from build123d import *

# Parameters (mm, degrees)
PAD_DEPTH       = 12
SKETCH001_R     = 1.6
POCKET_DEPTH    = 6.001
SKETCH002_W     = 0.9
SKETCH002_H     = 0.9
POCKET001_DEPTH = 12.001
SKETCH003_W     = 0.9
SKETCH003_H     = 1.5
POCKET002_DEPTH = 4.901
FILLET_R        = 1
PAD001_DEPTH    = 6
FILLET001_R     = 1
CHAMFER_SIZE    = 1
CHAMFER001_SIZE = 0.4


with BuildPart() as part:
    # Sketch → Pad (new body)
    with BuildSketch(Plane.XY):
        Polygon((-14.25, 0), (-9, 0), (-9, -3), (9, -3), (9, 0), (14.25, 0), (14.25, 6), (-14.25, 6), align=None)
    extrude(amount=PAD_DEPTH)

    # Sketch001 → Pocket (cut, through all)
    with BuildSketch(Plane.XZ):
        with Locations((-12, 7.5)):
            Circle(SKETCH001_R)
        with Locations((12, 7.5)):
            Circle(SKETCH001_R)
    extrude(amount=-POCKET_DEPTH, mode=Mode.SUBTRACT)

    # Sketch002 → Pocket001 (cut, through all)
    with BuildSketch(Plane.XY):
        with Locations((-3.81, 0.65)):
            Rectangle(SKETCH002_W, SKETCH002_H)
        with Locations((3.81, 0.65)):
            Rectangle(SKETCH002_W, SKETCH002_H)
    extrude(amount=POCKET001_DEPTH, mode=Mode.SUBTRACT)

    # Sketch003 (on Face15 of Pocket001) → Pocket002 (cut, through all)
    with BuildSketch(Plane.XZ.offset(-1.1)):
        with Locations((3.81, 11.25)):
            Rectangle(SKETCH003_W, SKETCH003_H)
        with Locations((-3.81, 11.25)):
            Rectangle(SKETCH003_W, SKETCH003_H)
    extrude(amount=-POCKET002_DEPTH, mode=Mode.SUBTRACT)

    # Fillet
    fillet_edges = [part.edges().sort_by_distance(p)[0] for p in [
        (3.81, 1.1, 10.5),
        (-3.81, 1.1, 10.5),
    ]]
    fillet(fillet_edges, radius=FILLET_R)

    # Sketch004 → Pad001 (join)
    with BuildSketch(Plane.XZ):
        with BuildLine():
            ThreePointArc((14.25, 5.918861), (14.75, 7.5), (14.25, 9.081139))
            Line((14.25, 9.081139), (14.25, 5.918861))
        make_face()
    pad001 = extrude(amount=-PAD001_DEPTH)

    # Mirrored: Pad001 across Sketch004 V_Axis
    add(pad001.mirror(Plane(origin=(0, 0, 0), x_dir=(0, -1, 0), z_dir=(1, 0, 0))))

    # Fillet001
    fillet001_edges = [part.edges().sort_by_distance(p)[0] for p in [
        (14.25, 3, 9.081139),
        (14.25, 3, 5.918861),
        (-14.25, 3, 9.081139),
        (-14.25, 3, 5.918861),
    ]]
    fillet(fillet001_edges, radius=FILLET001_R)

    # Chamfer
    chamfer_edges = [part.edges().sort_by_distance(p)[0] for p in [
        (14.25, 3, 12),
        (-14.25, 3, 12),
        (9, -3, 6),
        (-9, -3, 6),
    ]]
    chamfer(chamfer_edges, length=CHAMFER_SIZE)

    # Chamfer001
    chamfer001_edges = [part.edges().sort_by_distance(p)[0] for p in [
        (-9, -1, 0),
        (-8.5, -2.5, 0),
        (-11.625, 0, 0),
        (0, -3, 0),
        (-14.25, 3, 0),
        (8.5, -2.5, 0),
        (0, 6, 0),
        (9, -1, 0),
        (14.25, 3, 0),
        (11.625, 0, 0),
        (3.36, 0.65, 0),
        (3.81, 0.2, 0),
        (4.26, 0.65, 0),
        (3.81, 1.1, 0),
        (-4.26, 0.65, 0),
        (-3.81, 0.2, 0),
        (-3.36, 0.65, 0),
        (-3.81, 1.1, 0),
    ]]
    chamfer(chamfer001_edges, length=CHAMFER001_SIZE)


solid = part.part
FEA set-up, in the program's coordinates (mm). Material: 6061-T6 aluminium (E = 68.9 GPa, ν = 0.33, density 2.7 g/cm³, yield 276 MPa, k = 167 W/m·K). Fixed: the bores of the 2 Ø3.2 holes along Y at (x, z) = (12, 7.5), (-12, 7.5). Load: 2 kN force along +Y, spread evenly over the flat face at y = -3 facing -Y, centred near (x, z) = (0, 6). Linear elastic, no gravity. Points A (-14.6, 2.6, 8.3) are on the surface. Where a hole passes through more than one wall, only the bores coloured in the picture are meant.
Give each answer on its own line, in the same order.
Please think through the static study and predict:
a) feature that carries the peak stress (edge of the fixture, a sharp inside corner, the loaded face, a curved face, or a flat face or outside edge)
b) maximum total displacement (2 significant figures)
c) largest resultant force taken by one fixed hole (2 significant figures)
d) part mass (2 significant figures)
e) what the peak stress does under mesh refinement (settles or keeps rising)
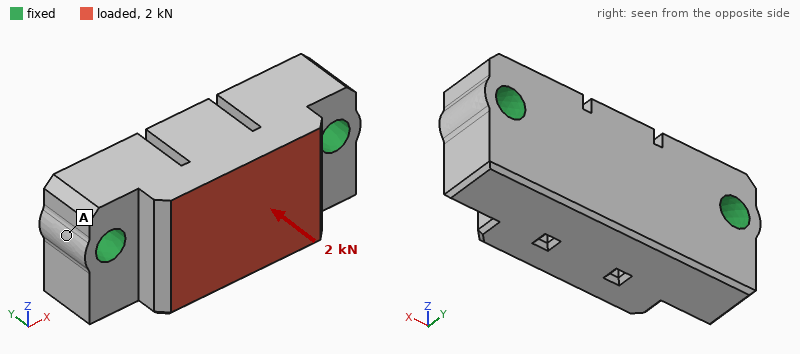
edge of the fixture
11 µm
1.1 kN
6.9 g
keeps rising
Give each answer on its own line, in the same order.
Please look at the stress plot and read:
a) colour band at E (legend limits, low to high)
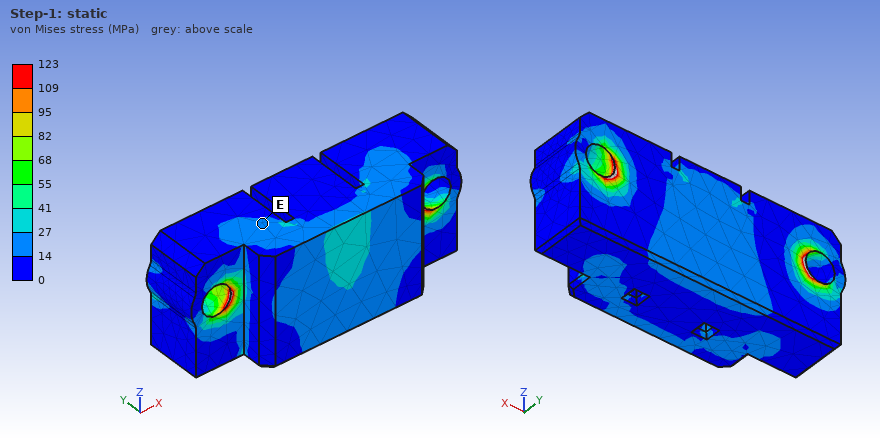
14 to 27 MPa
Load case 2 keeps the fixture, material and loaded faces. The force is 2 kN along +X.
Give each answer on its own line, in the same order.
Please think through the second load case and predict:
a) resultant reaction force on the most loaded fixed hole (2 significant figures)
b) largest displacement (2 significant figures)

1.1 kN
4.6 µm
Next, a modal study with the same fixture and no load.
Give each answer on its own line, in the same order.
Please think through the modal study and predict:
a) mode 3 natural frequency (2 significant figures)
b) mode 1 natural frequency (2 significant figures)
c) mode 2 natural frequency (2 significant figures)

47 kHz
32 kHz
40 kHz
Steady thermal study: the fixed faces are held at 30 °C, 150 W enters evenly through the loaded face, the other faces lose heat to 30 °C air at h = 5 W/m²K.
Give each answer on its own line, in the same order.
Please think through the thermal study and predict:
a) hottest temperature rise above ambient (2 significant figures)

64 K
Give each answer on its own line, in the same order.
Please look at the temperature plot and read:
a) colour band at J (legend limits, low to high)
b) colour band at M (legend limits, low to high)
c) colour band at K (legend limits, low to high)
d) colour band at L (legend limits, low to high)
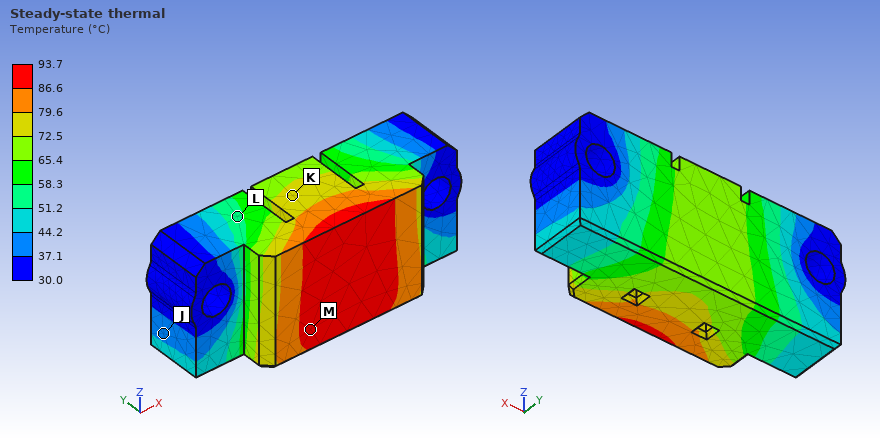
37.1 to 44.2 °C
86.6 to 93.7 °C
72.5 to 79.6 °C
51.2 to 58.3 °C
